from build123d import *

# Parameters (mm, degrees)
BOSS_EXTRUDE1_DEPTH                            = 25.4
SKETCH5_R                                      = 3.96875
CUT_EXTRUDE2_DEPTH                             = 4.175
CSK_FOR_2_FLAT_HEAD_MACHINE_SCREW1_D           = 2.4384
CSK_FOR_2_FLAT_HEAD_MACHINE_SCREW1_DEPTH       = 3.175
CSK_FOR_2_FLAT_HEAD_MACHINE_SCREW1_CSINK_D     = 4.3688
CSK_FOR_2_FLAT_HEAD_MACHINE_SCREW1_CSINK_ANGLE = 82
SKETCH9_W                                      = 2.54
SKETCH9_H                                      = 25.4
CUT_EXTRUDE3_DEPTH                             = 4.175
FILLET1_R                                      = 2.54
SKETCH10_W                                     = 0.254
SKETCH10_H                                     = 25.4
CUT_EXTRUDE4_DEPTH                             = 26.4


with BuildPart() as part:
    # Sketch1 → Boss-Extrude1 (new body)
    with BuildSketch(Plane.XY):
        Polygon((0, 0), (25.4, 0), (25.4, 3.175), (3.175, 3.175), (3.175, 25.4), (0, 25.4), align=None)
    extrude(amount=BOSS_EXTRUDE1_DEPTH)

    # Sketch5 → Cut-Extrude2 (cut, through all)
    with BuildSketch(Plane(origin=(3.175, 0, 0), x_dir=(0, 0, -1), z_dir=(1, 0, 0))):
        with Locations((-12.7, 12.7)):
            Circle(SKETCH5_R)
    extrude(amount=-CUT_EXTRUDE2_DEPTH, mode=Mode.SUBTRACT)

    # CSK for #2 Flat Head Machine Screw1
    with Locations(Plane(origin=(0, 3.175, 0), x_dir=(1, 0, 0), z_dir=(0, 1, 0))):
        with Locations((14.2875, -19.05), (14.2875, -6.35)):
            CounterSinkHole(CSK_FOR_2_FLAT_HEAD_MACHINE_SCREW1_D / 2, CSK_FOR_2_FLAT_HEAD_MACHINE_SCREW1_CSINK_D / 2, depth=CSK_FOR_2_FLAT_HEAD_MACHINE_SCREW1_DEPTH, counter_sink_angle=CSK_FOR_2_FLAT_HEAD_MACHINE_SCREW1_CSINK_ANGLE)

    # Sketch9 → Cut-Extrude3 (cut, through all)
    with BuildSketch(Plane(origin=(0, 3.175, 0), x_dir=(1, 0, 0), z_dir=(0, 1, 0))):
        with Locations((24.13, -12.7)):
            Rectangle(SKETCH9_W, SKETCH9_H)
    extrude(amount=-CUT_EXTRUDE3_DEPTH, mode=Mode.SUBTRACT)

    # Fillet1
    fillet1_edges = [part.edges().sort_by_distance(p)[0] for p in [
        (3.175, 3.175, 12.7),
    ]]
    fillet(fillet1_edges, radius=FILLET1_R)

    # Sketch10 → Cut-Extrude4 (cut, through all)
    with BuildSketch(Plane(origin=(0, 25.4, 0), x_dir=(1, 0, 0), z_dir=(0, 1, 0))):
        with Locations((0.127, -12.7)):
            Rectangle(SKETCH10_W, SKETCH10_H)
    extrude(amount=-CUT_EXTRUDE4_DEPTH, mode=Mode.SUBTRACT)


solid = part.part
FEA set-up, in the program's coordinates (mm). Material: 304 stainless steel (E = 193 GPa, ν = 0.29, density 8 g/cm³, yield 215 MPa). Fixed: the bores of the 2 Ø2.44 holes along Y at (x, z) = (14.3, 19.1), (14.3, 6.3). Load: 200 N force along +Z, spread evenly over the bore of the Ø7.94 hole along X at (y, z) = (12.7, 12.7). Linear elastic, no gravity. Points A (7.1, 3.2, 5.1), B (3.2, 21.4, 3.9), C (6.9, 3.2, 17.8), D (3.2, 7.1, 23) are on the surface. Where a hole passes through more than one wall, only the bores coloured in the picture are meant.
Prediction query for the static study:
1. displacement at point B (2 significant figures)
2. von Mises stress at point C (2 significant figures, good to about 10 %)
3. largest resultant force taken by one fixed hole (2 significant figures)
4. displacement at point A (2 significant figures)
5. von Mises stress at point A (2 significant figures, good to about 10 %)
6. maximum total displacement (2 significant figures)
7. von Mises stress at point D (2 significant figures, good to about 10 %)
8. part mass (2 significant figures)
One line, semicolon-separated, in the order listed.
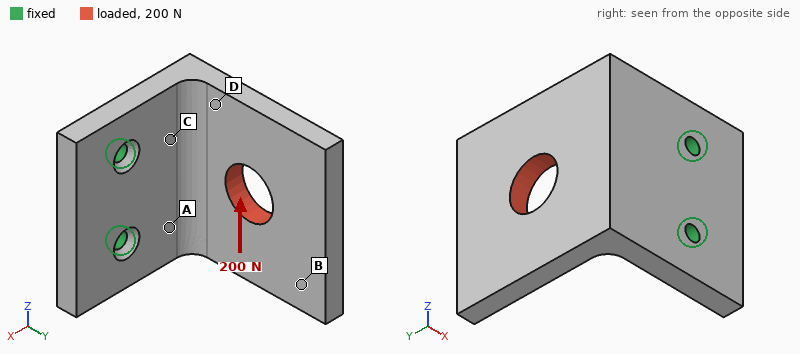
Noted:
17 µm; 31 MPa; 260 N; 3.4 µm; 26 MPa; 21 µm; 17 MPa; 27 g
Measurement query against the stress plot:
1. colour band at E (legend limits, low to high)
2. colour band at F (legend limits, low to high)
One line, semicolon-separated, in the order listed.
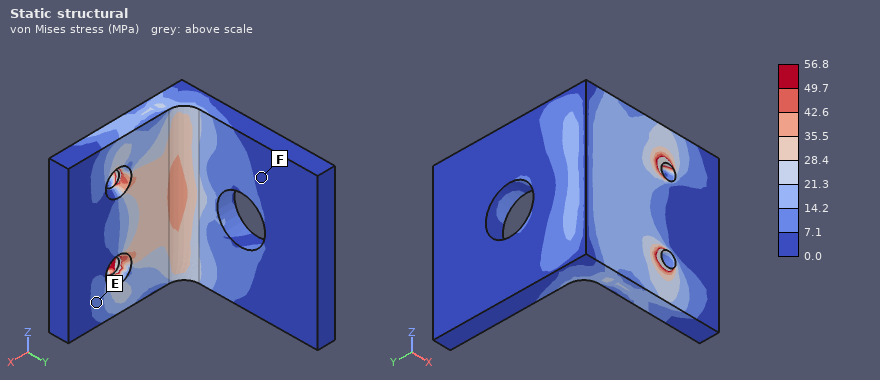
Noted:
7.1 to 14.2 MPa; 0.0 to 7.1 MPa
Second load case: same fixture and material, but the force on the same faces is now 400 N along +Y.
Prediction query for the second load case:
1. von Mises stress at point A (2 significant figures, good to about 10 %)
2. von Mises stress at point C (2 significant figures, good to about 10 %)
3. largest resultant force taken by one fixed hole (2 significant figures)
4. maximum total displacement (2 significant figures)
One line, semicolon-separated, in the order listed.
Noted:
42 MPa; 42 MPa; 200 N; 84 µm
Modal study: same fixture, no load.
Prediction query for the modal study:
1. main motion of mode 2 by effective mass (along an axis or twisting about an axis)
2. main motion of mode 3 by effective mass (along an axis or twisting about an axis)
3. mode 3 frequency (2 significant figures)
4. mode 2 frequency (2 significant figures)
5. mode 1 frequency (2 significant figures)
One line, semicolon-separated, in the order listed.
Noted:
along Z; along Y; 7200 Hz; 4600 Hz; 2400 Hz
